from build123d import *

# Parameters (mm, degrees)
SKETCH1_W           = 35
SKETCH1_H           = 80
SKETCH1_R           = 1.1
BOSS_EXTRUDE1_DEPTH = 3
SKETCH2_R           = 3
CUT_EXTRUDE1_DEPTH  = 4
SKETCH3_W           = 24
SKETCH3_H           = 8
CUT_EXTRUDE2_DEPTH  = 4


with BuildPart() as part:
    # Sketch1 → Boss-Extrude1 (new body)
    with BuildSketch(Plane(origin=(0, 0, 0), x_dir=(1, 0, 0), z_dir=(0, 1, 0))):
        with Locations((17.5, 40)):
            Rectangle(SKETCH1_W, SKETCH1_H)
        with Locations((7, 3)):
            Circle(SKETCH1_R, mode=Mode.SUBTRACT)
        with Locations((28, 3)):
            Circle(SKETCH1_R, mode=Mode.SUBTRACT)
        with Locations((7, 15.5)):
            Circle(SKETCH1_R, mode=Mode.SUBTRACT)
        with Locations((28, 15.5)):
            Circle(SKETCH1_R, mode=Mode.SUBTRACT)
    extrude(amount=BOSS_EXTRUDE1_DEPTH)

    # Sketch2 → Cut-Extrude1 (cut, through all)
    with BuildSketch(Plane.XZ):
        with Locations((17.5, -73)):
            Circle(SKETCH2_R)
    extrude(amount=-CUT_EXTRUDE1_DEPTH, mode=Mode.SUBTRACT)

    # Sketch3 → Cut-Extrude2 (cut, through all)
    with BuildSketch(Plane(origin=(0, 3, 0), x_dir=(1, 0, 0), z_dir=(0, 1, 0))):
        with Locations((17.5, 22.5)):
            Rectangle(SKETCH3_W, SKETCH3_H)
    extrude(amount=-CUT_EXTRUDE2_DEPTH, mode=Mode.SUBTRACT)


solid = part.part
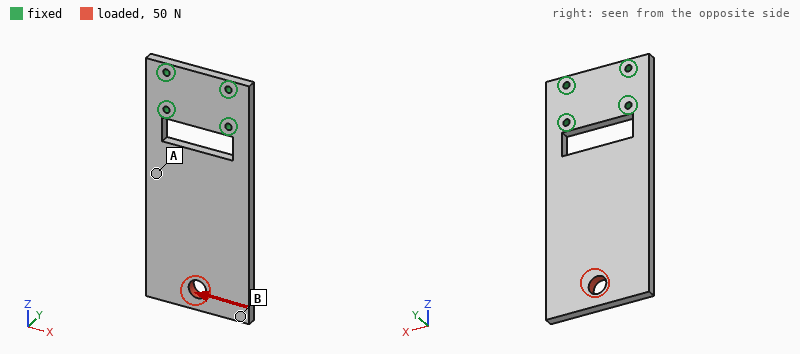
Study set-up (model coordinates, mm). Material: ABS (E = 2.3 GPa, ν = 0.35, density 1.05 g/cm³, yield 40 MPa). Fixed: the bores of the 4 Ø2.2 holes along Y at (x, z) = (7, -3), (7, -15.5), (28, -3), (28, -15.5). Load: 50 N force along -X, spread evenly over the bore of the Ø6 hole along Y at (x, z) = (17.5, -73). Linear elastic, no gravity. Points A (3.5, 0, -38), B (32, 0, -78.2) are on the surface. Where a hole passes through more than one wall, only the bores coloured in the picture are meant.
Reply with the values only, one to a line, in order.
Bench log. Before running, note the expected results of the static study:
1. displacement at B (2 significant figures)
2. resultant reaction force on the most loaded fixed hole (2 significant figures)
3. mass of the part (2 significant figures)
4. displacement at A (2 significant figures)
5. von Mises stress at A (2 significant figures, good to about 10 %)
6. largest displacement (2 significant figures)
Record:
0.39 mm
76 N
8.1 g
0.17 mm
2.4 MPa
0.40 mm
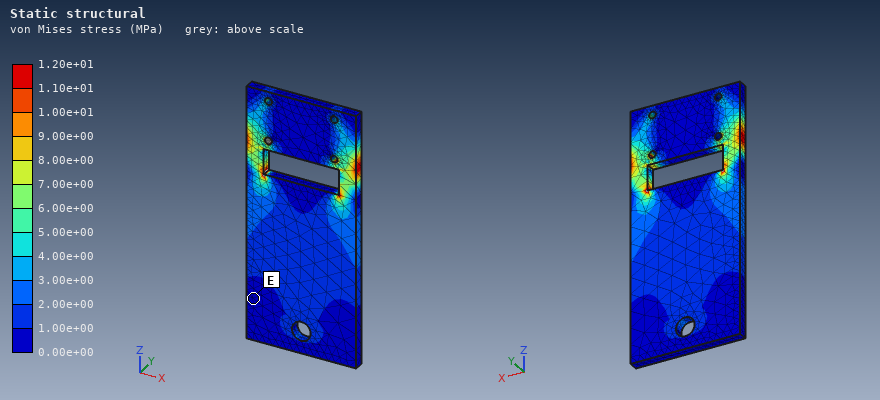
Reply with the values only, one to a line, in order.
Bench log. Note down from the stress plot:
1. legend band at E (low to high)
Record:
0.00e+00 to 1.00e+00 MPa
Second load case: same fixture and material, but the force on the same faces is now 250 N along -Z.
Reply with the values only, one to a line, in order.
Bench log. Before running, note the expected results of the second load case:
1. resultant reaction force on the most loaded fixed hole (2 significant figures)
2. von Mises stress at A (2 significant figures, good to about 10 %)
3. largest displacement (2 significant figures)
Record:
94 N
4.1 MPa
0.15 mm
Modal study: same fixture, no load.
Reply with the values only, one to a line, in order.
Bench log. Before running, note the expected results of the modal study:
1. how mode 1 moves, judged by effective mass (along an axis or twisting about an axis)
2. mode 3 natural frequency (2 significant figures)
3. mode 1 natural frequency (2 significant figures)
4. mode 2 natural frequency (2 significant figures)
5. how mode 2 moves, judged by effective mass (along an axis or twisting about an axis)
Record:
along Y
920 Hz
110 Hz
590 Hz
twisting about Z
